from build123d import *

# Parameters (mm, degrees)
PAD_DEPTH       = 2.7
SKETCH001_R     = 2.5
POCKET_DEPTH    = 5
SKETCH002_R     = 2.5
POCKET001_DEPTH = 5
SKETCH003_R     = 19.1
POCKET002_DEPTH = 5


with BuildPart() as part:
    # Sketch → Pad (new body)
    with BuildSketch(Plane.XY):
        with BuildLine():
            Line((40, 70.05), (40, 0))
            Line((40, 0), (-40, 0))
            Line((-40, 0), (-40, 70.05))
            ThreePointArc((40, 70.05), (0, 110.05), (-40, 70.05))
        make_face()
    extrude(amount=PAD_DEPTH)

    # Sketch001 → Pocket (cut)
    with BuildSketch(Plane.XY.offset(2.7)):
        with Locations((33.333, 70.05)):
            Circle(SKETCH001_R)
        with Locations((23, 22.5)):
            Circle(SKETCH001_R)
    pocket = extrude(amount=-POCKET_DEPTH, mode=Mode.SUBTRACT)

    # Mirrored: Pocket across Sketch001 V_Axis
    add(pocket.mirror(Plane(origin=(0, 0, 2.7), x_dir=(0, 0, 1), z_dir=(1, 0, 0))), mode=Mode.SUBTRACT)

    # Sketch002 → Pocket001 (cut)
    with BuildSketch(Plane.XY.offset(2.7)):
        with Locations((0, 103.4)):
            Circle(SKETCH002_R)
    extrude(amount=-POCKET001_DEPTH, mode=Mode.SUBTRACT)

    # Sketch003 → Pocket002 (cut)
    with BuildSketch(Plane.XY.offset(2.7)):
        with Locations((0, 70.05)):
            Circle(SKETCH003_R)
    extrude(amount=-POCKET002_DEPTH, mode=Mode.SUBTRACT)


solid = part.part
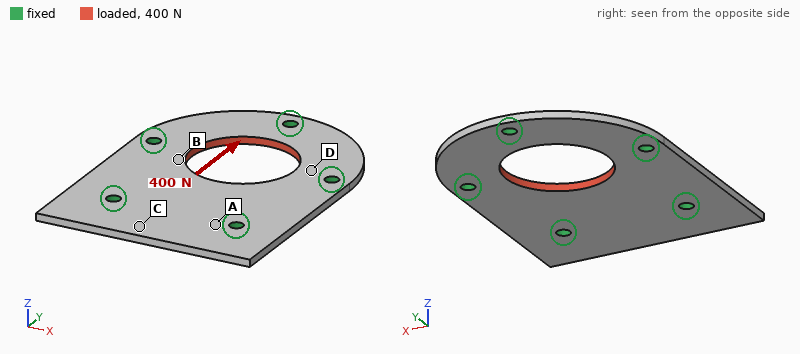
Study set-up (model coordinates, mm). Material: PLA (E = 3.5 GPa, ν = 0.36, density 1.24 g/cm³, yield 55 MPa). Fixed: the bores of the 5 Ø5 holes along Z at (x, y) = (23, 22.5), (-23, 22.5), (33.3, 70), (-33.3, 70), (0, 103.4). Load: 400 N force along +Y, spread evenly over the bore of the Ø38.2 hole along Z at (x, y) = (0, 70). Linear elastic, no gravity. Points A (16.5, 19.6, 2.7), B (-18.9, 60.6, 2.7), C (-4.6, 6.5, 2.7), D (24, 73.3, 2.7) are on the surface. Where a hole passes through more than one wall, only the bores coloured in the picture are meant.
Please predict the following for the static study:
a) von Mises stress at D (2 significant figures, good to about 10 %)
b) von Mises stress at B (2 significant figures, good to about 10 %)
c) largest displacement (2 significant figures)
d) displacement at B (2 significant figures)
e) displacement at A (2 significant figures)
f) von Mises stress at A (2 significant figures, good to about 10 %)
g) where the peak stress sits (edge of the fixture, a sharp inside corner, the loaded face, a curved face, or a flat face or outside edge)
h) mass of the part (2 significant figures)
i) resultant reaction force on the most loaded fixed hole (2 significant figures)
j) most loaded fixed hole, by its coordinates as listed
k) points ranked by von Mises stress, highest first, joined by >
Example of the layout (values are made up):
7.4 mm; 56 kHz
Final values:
1.2 MPa; 1.7 MPa; 16 µm; 12 µm; 2.8 µm; 0.72 MPa; edge of the fixture; 23 g; 99 N; (0, 103.4); B > D > A > C
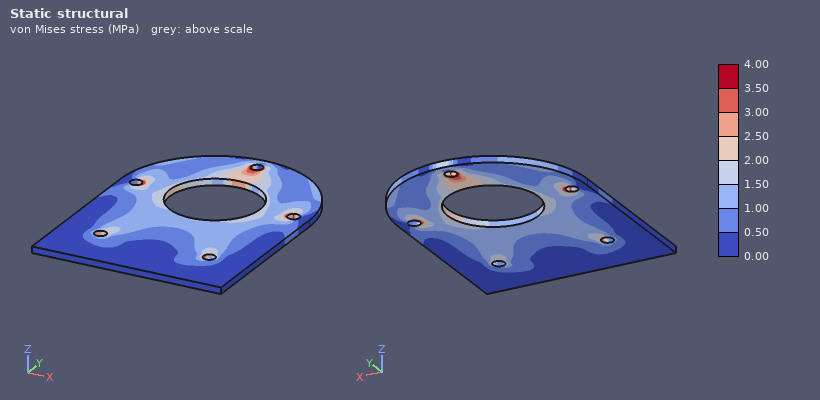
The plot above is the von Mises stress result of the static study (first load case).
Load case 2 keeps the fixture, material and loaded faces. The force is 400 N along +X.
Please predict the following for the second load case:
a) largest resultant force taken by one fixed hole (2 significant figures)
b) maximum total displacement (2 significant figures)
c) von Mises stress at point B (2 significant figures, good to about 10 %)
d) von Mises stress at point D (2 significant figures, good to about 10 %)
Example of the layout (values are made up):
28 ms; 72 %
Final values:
110 N; 18 µm; 1.6 MPa; 2.2 MPa
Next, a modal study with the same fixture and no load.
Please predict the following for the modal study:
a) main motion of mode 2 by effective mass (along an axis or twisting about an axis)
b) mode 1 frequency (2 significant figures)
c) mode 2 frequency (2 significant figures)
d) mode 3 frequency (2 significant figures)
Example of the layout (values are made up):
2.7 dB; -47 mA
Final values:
along Z; 1200 Hz; 1400 Hz; 1600 Hz
